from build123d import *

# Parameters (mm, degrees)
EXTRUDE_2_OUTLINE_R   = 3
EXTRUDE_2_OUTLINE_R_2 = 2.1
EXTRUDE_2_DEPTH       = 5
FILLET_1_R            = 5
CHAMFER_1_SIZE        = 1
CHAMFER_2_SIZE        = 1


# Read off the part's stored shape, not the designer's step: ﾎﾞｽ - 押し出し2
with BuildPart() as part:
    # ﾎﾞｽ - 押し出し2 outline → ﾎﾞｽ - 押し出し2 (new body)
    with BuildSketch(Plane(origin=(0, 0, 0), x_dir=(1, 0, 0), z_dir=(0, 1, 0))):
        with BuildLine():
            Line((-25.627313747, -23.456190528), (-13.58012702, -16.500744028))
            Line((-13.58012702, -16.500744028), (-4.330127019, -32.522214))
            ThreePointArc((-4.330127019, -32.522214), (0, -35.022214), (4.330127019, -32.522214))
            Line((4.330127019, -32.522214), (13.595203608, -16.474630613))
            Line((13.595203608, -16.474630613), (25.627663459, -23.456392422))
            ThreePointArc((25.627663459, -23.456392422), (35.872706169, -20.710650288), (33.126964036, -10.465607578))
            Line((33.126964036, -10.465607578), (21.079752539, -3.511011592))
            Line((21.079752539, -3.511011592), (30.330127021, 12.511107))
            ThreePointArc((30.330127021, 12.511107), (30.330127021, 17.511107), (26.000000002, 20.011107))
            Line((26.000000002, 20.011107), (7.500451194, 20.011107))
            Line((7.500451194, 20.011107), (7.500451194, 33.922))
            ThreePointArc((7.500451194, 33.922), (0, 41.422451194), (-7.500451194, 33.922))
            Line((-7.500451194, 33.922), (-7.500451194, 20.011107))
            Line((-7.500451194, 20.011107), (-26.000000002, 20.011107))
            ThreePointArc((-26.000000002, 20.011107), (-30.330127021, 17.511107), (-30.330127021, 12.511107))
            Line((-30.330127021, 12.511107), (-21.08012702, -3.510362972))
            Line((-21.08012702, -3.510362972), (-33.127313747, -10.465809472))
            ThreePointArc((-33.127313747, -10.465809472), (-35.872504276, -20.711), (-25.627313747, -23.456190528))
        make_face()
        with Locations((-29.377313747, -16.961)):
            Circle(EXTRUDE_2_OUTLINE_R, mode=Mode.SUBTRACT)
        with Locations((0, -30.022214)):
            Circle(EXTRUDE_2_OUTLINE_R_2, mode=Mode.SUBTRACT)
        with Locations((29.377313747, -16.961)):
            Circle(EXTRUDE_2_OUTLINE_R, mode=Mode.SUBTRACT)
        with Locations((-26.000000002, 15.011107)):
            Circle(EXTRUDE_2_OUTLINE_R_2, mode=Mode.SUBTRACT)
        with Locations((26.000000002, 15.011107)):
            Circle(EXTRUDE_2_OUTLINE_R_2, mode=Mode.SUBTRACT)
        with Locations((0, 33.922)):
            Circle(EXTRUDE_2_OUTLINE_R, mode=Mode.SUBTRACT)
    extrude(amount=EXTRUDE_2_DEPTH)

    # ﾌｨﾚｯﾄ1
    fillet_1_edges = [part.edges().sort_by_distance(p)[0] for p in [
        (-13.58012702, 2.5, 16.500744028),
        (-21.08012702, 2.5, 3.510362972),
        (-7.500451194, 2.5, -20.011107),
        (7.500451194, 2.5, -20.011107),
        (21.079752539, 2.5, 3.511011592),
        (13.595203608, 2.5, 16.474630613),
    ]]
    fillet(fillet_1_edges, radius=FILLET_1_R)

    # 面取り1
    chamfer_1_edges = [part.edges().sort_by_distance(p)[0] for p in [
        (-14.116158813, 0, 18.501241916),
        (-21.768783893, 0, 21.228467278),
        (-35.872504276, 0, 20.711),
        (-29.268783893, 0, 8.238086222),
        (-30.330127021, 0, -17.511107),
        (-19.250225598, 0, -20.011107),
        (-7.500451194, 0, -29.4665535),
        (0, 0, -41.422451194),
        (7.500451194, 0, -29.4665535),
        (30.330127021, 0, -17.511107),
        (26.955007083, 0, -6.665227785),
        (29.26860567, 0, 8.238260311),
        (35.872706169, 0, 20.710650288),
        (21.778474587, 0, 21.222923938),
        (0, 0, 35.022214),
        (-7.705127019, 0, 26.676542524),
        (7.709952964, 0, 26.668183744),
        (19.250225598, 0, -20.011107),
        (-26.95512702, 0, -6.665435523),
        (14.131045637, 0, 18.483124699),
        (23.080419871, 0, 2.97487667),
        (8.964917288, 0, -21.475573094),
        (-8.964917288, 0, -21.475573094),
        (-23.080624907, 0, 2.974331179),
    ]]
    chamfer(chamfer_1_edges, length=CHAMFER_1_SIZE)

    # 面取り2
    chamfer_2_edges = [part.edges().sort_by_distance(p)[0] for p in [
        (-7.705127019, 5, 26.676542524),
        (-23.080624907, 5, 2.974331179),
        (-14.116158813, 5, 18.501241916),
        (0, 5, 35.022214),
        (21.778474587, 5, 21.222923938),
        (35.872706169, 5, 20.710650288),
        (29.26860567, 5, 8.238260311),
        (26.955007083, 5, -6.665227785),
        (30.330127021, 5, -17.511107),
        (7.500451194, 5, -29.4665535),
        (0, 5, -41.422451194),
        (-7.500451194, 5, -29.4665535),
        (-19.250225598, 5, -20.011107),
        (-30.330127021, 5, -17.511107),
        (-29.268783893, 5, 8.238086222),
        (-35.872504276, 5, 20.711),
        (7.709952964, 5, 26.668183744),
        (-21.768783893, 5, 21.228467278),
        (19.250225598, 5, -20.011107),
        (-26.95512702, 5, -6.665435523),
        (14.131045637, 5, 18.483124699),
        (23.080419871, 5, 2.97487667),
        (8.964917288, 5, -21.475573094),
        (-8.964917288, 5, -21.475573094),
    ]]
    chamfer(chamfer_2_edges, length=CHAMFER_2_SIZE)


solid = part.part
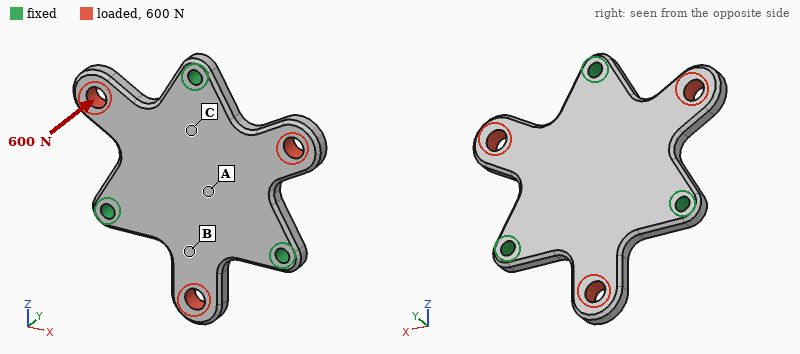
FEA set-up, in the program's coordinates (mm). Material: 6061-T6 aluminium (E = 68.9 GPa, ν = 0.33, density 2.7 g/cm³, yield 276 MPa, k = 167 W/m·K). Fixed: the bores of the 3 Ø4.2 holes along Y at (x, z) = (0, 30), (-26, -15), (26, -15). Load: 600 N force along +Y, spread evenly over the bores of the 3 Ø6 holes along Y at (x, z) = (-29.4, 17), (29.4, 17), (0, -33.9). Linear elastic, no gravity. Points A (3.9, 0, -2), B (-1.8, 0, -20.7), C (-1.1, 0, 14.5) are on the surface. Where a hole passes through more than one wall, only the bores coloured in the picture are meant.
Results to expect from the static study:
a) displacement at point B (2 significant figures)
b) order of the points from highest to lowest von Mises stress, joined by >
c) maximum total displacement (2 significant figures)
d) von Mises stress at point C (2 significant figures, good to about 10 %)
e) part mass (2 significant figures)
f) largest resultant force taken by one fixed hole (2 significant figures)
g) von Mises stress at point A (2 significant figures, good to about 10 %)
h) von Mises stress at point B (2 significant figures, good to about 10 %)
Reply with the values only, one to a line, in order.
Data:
0.025 mm
B > C > A
0.11 mm
22 MPa
37 g
200 N
13 MPa
38 MPa
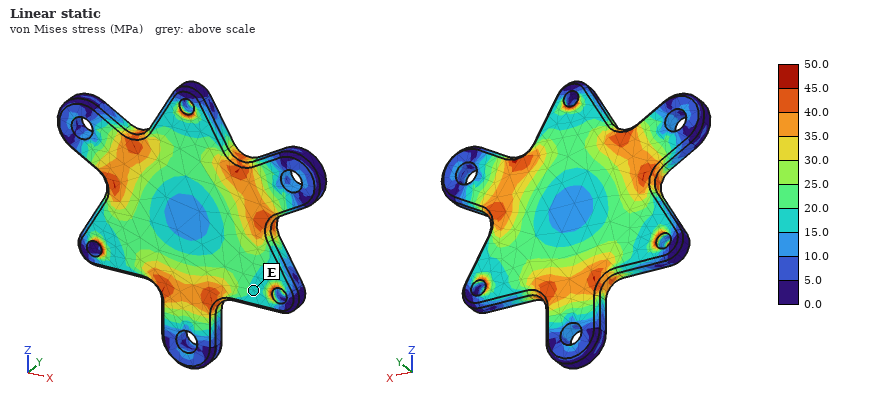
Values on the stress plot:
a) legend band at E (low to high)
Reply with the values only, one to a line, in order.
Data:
15.0 to 20.0 MPa
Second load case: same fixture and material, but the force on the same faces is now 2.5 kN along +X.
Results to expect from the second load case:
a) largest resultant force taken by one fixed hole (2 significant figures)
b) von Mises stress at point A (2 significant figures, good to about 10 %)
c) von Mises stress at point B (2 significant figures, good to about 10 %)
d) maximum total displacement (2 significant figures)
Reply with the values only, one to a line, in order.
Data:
920 N
15 MPa
6.5 MPa
37 µm
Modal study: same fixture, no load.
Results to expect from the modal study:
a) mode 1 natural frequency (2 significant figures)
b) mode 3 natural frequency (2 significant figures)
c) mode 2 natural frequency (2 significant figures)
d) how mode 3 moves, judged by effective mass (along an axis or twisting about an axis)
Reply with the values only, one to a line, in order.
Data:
4400 Hz
5100 Hz
4400 Hz
along Y
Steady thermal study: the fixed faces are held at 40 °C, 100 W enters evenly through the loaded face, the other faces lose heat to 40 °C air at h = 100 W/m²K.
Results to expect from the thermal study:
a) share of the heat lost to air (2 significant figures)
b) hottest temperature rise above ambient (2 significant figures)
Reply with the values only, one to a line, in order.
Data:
23 %
80 K
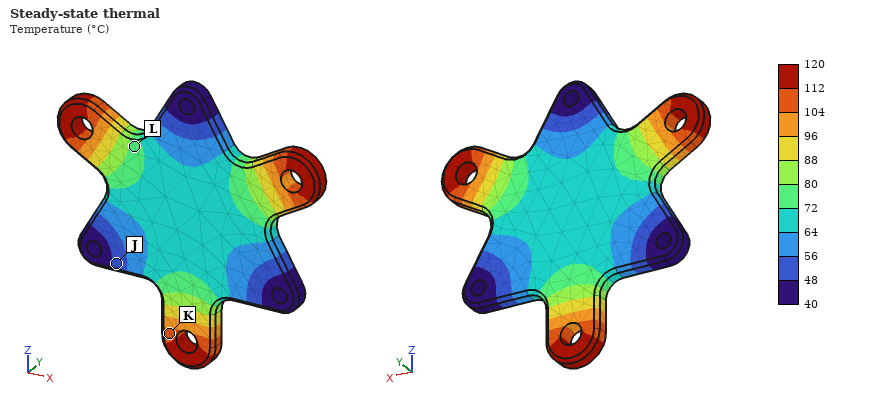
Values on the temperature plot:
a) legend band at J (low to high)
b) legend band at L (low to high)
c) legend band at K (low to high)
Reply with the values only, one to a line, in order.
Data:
48 to 56 °C
72 to 80 °C
104 to 112 °C
